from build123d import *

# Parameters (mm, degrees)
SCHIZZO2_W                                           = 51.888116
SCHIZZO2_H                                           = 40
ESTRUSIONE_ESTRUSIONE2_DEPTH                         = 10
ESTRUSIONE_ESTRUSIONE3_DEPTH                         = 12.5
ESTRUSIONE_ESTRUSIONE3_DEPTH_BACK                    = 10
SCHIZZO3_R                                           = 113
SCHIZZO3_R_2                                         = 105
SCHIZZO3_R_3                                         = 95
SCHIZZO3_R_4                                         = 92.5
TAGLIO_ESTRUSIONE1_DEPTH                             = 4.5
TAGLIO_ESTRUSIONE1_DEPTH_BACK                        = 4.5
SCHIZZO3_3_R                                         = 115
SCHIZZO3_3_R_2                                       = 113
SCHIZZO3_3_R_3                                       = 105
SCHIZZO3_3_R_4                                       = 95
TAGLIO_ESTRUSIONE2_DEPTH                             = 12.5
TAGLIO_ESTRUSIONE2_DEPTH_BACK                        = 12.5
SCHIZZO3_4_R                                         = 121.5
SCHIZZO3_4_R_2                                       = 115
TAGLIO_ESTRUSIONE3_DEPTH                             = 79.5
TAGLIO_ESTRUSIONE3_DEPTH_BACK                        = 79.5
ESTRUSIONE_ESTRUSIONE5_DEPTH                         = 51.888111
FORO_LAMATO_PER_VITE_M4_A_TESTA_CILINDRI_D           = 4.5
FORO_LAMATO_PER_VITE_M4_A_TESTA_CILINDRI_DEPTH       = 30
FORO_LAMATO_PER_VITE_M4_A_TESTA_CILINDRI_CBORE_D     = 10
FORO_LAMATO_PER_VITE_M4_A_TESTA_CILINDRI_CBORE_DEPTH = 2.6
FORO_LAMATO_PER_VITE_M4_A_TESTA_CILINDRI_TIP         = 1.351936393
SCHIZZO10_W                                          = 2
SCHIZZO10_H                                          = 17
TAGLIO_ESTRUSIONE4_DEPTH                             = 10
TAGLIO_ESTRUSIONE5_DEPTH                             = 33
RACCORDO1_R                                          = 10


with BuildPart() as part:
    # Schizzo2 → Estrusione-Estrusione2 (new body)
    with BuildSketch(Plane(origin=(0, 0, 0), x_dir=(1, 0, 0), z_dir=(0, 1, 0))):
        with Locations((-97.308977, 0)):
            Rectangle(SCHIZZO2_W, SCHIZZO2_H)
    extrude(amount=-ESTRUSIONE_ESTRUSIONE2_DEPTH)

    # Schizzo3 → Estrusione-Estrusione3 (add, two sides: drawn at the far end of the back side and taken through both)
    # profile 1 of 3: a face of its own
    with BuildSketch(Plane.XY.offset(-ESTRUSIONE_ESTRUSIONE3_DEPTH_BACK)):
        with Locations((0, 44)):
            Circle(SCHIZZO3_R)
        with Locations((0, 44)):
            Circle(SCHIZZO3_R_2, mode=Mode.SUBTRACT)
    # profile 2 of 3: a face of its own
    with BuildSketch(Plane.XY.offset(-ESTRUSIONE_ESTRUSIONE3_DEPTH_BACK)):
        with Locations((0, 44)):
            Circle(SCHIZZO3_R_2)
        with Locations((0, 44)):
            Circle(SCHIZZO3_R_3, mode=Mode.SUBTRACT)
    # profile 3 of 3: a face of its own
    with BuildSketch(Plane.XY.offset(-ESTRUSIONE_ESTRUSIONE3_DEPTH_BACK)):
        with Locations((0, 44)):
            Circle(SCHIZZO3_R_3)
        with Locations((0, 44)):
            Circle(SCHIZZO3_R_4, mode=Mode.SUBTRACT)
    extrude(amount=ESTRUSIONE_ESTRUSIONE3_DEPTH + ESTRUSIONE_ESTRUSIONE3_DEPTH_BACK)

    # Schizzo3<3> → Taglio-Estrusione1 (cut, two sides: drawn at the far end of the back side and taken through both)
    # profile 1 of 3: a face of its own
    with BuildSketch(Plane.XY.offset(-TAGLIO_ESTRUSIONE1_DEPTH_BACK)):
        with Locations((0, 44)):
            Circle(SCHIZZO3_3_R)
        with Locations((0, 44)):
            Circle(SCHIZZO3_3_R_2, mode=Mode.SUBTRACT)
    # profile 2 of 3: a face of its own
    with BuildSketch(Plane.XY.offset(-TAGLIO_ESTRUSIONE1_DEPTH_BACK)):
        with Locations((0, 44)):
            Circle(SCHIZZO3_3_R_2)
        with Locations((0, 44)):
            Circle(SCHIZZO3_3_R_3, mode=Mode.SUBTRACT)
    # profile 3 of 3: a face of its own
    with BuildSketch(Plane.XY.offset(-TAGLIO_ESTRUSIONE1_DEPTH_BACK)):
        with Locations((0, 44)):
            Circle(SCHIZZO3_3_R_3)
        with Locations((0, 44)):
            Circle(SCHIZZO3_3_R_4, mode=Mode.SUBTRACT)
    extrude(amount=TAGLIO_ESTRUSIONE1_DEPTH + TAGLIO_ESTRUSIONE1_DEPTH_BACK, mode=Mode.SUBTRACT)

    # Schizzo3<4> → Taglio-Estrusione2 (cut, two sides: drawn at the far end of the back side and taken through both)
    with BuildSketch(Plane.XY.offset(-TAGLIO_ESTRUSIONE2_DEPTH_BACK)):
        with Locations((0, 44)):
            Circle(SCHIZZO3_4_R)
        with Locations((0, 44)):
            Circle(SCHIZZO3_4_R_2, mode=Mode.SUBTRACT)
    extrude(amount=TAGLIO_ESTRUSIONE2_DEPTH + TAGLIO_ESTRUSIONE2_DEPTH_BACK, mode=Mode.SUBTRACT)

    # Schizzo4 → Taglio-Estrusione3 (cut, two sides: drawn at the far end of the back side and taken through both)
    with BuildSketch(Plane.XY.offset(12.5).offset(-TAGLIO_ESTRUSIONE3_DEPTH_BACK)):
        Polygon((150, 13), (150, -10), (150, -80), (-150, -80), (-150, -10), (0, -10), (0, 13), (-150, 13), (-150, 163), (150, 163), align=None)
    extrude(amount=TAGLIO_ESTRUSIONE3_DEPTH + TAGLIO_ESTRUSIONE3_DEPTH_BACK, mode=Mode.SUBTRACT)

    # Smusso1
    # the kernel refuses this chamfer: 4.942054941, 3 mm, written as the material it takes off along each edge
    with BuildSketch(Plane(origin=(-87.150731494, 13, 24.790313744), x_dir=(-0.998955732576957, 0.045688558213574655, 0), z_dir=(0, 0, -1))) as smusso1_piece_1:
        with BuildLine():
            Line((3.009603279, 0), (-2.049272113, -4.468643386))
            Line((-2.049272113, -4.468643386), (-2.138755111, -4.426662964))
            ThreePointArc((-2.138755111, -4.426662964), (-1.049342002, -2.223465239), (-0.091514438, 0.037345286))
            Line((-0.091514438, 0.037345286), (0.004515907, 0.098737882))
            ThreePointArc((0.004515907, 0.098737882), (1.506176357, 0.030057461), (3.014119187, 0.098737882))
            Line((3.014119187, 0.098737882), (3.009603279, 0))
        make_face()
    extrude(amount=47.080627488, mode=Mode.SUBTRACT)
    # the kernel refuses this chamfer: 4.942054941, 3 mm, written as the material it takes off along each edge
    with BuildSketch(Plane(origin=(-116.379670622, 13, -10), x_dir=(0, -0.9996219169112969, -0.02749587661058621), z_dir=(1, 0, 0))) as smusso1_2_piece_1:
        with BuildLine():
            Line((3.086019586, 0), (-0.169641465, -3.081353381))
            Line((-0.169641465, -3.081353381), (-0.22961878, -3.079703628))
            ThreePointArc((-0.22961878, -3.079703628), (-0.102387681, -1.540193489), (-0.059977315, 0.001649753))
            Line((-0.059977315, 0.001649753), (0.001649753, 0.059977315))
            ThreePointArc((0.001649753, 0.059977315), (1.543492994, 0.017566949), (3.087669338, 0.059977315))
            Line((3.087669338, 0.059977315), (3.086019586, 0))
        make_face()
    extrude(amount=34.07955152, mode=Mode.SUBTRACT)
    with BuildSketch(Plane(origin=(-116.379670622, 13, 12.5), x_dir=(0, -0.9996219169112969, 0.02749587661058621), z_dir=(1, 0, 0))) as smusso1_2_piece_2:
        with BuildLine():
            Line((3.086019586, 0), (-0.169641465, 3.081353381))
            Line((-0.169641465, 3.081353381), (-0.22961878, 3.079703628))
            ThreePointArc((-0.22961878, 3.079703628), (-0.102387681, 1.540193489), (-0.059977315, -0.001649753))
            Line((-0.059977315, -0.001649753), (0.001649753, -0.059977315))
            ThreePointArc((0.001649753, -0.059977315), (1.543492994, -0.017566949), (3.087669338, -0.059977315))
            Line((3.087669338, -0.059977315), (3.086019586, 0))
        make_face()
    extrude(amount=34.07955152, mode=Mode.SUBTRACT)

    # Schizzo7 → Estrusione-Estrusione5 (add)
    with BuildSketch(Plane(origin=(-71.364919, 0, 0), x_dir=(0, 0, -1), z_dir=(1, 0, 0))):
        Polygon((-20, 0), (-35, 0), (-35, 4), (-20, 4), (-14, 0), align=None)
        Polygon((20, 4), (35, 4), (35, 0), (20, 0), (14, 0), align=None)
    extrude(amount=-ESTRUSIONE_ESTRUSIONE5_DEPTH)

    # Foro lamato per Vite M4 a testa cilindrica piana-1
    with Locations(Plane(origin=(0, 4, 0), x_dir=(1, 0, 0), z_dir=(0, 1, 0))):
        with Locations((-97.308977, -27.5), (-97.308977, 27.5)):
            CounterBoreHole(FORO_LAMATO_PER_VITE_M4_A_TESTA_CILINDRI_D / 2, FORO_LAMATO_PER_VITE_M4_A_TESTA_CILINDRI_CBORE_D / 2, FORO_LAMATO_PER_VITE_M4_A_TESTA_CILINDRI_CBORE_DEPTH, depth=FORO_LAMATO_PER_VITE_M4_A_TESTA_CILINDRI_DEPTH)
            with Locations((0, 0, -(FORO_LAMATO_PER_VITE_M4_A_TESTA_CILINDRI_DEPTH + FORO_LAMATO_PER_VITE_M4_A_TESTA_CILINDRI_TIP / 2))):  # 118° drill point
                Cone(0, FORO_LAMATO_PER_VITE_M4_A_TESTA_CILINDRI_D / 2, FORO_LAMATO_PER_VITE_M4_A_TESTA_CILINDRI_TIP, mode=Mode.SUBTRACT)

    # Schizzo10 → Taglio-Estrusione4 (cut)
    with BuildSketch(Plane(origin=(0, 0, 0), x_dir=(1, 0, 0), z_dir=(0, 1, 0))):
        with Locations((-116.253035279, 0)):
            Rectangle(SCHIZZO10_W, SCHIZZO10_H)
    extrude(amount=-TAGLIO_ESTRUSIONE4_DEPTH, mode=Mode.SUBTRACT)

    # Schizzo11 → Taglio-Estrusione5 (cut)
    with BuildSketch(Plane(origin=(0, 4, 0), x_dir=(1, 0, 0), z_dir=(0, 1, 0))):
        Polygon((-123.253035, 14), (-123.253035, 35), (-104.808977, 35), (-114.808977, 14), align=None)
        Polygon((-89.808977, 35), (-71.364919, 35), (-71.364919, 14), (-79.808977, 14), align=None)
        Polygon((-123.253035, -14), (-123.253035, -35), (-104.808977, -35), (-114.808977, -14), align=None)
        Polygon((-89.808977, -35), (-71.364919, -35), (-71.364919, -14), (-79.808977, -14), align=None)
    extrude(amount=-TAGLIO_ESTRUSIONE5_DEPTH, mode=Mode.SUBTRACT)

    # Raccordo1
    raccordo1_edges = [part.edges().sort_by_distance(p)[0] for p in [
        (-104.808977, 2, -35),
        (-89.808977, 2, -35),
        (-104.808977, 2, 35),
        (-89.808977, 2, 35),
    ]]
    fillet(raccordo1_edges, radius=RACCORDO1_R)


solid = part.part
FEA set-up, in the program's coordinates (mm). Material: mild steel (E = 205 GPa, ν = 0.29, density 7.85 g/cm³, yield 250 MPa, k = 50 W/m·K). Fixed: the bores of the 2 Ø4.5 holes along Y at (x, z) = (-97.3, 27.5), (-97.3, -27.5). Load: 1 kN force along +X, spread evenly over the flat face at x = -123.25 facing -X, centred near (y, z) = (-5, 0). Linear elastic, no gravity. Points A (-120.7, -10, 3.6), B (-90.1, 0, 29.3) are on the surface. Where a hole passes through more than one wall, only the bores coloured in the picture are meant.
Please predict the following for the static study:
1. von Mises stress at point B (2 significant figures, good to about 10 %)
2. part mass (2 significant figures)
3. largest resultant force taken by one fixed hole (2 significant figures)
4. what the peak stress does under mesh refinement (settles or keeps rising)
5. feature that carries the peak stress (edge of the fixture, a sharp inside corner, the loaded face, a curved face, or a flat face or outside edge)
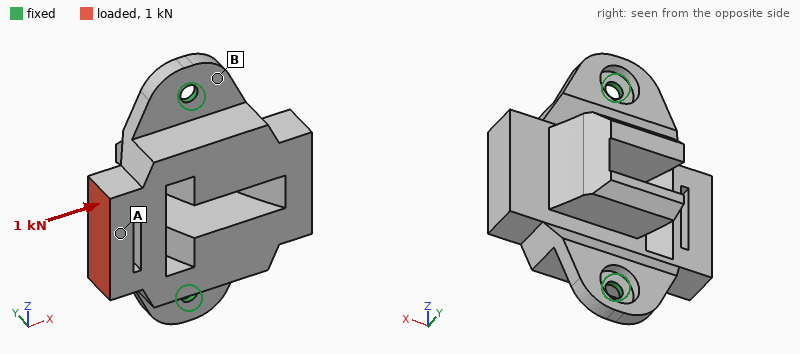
38 MPa
160 g
500 N
keeps rising
edge of the fixture
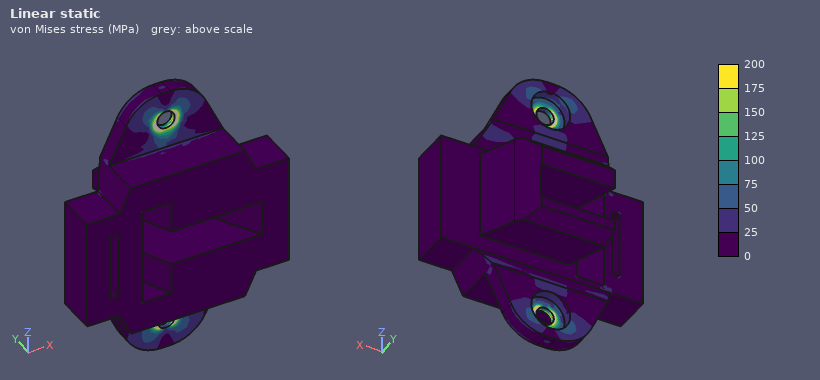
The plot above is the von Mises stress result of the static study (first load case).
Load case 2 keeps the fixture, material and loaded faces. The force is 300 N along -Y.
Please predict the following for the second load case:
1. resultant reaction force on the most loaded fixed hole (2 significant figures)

220 N
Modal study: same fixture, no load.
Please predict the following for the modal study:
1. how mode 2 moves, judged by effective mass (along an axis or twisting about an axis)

along Y
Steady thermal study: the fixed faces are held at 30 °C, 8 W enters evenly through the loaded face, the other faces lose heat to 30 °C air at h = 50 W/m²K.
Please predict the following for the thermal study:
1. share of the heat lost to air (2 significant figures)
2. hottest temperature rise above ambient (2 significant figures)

54 %
32 K
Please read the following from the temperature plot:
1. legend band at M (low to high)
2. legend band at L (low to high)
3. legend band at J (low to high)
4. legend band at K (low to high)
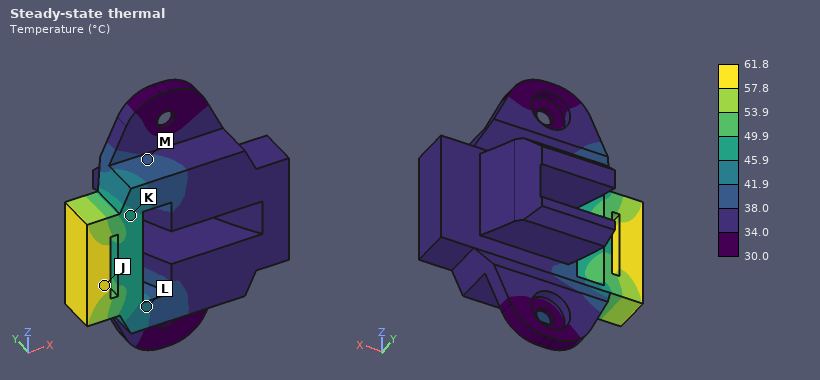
38.0 to 41.9 °C
41.9 to 45.9 °C
57.8 to 61.8 °C
45.9 to 49.9 °C
